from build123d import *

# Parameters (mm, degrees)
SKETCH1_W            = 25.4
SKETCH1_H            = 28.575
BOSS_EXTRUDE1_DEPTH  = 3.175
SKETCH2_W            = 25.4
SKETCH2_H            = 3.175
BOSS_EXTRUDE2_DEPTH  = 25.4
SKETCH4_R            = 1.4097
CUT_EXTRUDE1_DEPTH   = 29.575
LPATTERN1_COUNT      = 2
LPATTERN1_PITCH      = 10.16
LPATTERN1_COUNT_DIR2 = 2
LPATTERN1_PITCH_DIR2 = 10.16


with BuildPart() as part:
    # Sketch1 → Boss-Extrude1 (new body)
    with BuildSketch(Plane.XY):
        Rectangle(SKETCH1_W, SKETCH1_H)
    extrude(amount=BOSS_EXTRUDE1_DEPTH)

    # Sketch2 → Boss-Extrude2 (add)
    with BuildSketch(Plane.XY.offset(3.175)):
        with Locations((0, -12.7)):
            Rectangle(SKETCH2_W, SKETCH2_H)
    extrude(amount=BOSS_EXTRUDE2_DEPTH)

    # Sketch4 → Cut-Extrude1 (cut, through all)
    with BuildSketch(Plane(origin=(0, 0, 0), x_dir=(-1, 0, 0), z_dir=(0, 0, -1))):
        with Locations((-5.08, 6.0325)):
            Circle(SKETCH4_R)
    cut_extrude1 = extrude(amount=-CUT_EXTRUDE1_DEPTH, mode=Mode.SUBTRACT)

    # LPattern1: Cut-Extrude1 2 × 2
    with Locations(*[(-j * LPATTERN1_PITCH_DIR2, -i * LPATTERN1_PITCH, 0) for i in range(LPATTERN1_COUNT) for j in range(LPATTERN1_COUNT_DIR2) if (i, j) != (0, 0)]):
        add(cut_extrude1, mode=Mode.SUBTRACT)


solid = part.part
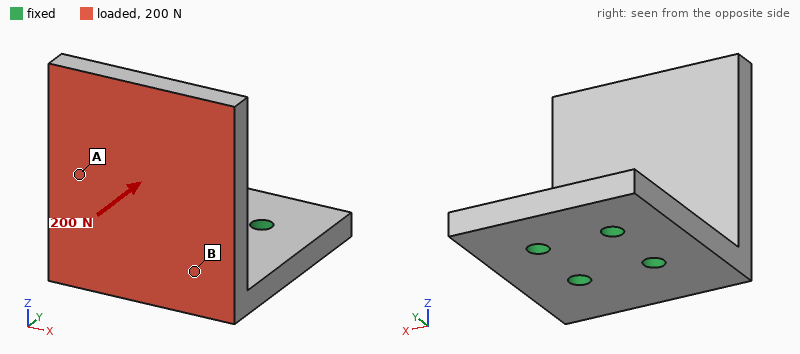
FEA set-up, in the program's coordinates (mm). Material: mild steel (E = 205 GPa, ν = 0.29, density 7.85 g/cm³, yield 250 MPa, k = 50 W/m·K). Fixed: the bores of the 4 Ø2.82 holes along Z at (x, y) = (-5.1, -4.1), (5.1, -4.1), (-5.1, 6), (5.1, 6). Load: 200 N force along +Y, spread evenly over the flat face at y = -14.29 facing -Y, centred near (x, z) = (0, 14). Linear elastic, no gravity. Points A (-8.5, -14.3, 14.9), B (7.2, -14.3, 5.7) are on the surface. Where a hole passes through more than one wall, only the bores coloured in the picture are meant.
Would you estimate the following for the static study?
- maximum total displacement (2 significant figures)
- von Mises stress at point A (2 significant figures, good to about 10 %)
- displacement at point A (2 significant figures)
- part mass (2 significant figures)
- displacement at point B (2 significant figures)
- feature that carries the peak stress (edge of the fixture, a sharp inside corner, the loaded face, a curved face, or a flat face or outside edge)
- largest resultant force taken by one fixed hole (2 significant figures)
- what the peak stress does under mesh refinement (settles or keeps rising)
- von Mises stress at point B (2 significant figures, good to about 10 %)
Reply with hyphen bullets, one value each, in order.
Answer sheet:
- 68 µm
- 15 MPa
- 30 µm
- 34 g
- 12 µm
- edge of the fixture
- 96 N
- keeps rising
- 40 MPa
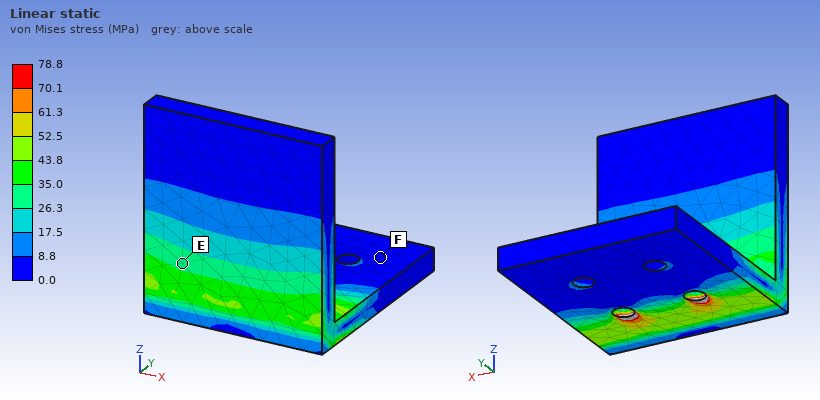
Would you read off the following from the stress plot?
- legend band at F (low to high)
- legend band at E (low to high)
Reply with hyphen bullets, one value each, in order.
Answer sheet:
- 0.0 to 8.8 MPa
- 26.3 to 35.0 MPa
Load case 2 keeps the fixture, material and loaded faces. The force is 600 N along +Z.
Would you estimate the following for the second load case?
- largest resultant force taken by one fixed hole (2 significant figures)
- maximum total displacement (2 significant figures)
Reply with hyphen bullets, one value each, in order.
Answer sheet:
- 370 N
- 72 µm
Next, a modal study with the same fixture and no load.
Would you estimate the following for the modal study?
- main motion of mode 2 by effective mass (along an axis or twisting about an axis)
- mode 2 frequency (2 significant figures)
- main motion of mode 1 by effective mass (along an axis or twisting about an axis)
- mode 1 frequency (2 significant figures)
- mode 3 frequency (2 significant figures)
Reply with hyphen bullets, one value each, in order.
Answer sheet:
- along X
- 5200 Hz
- along Y
- 2500 Hz
- 8600 Hz
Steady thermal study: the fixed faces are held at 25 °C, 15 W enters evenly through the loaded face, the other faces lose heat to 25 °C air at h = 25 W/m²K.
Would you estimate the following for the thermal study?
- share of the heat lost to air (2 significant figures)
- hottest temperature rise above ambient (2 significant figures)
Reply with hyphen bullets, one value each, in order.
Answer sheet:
- 10 %
- 69 K
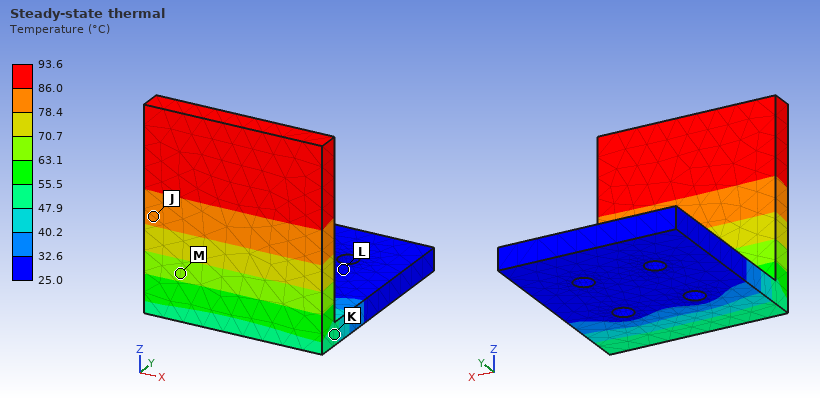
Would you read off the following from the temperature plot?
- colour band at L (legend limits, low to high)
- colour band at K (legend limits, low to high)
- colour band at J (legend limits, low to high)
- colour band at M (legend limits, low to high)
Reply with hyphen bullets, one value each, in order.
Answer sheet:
- 25.0 to 32.6 °C
- 47.9 to 55.5 °C
- 78.4 to 86.0 °C
- 63.1 to 70.7 °C
